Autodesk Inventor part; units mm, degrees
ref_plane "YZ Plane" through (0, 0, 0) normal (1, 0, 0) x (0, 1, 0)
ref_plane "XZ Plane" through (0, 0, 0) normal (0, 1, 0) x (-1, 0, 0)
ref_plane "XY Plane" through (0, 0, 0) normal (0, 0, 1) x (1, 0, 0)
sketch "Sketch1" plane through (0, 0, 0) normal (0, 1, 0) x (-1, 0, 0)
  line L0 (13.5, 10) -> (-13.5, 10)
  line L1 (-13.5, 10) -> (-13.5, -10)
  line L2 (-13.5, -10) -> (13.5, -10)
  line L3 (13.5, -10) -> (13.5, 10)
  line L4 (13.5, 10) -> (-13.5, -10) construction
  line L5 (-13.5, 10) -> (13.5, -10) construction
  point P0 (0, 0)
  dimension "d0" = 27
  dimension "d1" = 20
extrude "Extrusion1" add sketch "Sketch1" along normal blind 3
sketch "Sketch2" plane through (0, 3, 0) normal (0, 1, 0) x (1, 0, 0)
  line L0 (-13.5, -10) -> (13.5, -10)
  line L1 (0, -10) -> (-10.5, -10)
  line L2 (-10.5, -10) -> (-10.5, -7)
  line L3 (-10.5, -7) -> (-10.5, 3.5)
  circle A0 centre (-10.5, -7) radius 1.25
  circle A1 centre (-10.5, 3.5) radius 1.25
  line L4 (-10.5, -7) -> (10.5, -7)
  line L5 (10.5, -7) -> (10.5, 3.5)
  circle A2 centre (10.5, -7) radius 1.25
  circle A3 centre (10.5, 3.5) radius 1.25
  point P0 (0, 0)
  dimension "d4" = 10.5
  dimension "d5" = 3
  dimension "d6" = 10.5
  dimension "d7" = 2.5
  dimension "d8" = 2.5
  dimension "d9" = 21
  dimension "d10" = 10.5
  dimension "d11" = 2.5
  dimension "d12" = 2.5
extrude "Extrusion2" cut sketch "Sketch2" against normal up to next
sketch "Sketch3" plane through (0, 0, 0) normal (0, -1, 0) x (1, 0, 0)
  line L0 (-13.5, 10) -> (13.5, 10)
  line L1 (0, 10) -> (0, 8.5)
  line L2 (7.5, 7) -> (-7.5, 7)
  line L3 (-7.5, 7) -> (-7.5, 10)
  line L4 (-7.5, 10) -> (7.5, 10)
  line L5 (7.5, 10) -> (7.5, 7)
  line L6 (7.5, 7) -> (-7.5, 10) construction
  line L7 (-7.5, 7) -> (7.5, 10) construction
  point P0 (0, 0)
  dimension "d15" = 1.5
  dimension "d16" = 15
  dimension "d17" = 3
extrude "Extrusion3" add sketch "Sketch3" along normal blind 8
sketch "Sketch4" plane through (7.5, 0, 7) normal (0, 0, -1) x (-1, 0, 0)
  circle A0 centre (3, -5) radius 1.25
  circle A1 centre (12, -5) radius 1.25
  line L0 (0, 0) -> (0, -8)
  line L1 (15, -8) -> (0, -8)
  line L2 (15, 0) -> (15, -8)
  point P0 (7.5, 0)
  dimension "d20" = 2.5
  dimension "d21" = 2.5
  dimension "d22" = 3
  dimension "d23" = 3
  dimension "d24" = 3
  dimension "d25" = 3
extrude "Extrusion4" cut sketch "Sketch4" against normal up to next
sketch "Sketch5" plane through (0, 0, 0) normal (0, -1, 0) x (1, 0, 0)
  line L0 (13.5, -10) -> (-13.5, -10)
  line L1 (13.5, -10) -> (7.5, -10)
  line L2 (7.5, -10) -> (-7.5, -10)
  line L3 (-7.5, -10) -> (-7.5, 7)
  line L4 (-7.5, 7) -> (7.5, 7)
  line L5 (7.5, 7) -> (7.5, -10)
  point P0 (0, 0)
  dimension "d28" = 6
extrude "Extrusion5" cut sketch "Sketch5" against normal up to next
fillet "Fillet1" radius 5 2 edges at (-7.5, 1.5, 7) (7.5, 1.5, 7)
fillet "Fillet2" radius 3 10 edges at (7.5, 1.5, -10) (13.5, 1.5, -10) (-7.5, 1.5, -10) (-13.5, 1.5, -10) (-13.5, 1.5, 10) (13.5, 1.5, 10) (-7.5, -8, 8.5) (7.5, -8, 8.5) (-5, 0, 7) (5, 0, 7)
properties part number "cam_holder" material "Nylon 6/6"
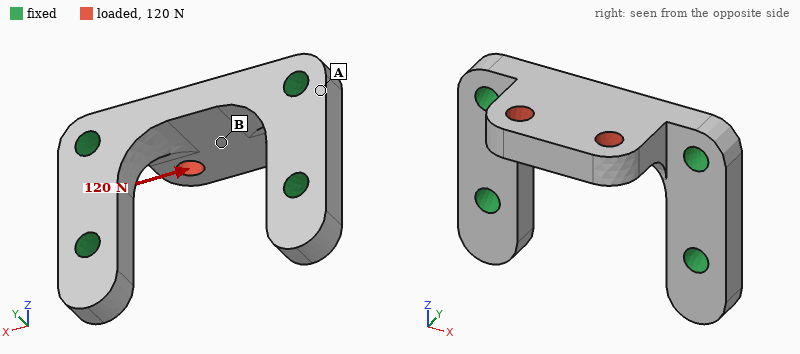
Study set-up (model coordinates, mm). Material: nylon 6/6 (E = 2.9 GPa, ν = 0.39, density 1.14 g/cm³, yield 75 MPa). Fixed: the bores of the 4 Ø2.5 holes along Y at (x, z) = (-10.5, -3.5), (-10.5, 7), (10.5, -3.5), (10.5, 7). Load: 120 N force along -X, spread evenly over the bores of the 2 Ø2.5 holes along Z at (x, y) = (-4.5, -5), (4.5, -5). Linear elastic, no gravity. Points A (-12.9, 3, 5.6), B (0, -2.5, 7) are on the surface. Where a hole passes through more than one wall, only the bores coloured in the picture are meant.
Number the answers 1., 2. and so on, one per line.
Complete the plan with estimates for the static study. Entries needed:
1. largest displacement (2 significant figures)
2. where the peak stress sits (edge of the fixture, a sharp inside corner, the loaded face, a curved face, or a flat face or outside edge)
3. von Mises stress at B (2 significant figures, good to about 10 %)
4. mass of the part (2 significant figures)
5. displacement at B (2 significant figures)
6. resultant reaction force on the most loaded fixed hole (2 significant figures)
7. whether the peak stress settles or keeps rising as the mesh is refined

1. 52 µm
2. edge of the fixture
3. 5.0 MPa
4. 1.3 g
5. 24 µm
6. 75 N
7. keeps rising
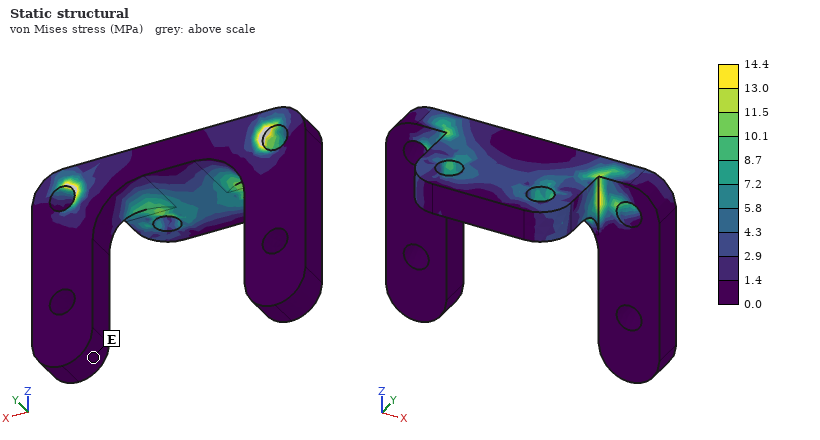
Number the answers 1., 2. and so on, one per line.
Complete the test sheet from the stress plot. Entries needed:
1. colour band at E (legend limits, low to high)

1. 0.0 to 1.4 MPa
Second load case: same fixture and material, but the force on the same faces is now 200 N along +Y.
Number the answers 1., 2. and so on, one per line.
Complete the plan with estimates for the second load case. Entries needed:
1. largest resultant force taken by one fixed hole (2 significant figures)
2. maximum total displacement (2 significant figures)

1. 110 N
2. 0.14 mm
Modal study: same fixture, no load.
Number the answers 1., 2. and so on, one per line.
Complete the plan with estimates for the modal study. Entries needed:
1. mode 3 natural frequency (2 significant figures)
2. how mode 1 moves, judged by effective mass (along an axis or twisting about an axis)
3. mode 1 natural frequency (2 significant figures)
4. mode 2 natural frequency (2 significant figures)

1. 13 kHz
2. along Z
3. 5700 Hz
4. 13 kHz
